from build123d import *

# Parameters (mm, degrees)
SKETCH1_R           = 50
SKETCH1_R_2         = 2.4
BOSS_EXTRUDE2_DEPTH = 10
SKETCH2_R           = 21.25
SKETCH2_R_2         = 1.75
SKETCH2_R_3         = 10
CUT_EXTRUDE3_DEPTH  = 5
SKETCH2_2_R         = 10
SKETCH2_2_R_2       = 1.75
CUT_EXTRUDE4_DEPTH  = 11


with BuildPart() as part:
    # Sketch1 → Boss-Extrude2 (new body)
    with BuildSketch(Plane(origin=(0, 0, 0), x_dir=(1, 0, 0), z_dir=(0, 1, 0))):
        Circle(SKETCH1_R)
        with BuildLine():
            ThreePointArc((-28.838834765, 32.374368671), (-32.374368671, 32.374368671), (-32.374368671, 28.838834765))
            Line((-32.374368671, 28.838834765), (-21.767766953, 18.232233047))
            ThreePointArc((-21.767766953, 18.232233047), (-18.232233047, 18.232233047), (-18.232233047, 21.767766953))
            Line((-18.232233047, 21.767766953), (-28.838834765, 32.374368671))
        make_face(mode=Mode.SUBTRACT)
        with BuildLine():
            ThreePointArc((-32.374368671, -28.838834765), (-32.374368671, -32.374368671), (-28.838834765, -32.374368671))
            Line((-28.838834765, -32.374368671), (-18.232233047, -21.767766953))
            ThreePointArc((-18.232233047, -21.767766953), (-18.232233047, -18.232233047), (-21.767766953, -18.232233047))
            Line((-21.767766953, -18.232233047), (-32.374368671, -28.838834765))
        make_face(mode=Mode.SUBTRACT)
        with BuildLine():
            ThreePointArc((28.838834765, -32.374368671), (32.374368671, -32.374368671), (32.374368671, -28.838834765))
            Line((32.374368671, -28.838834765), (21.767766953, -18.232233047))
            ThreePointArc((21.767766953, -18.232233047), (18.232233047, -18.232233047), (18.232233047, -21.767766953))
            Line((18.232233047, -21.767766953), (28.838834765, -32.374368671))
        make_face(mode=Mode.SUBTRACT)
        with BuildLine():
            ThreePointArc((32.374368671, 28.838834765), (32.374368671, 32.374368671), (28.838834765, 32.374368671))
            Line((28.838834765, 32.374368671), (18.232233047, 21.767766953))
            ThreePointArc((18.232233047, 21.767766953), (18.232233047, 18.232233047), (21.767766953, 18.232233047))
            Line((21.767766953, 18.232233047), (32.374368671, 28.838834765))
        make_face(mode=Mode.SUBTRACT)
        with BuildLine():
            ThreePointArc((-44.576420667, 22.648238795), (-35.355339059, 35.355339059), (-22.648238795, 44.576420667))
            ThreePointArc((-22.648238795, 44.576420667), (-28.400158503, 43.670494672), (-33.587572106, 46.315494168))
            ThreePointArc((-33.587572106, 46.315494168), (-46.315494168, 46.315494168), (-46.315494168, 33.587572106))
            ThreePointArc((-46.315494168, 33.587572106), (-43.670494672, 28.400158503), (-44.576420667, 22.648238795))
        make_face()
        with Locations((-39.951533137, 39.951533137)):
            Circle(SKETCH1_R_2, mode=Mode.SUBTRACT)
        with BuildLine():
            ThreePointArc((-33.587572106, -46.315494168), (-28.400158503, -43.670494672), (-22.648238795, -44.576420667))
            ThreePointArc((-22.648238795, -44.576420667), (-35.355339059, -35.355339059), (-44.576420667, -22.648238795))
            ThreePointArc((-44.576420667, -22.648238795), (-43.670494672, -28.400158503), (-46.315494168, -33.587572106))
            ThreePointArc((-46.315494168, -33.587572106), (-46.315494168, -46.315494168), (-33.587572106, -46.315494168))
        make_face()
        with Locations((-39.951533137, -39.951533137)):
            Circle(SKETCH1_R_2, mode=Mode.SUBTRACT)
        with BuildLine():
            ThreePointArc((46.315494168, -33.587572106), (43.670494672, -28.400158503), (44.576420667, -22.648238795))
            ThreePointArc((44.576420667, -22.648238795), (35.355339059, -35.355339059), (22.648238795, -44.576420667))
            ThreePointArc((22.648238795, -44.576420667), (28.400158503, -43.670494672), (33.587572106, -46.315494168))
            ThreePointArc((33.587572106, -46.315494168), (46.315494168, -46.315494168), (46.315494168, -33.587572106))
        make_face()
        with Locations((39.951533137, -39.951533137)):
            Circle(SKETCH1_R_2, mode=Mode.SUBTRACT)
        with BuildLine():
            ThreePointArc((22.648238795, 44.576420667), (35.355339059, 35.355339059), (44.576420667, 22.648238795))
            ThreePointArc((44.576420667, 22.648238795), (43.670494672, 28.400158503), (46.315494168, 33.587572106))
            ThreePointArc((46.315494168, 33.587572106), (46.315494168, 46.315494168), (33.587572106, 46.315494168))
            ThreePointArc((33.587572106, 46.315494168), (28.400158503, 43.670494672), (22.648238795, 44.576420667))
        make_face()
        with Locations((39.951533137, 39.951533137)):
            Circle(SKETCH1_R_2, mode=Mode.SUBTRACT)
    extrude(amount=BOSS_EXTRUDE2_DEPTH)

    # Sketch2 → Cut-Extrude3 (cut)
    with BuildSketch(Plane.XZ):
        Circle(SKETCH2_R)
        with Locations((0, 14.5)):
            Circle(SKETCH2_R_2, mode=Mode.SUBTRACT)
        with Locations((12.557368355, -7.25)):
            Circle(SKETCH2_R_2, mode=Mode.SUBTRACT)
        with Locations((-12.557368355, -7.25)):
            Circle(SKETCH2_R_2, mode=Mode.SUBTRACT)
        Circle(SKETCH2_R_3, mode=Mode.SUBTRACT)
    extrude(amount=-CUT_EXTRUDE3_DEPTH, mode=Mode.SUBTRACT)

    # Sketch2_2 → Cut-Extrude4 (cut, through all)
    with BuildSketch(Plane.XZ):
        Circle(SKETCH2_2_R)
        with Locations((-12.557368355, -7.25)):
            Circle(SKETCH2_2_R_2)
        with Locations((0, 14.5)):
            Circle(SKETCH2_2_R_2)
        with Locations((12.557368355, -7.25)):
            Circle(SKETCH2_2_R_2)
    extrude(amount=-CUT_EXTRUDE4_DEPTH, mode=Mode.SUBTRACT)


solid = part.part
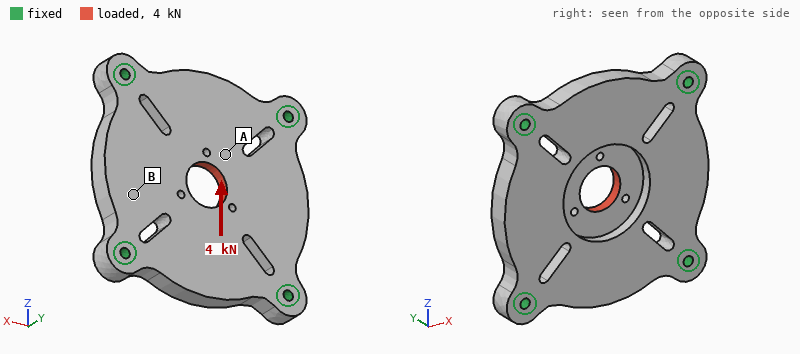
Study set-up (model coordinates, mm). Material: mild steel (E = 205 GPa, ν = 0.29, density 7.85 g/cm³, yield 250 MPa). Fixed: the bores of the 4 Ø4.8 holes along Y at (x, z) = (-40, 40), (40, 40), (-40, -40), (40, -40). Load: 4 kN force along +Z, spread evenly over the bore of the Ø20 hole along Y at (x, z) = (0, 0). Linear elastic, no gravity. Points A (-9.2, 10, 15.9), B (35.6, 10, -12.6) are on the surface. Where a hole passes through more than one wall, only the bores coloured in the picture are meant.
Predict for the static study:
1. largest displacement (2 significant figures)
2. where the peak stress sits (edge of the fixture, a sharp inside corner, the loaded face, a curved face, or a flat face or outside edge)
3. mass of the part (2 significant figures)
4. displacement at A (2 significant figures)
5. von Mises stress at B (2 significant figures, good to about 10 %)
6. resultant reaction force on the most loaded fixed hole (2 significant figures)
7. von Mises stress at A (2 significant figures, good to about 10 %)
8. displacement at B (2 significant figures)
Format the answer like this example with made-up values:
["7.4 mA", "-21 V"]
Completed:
["2.9 µm", "a curved face", "600 g", "2.1 µm", "2.7 MPa", "1.1 kN", "9.6 MPa", "0.64 µm"]
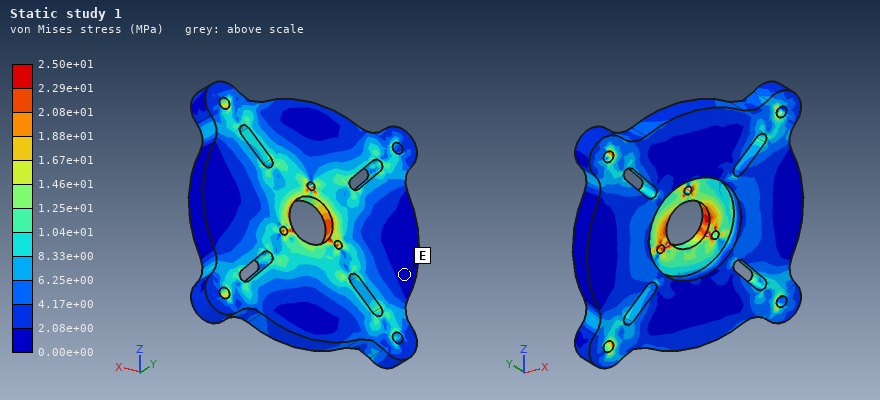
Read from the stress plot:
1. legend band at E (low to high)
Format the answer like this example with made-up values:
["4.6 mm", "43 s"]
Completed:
["0.00e+00 to 2.08e+00 MPa"]
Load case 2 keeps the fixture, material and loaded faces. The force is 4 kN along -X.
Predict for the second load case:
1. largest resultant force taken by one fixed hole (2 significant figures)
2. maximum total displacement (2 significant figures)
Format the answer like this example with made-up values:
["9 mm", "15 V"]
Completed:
["1.2 kN", "2.8 µm"]
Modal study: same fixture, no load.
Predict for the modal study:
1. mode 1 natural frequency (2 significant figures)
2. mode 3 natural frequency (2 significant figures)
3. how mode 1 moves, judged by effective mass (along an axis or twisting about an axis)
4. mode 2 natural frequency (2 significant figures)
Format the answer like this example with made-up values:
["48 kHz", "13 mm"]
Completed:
["4800 Hz", "7000 Hz", "along Y", "7000 Hz"]
